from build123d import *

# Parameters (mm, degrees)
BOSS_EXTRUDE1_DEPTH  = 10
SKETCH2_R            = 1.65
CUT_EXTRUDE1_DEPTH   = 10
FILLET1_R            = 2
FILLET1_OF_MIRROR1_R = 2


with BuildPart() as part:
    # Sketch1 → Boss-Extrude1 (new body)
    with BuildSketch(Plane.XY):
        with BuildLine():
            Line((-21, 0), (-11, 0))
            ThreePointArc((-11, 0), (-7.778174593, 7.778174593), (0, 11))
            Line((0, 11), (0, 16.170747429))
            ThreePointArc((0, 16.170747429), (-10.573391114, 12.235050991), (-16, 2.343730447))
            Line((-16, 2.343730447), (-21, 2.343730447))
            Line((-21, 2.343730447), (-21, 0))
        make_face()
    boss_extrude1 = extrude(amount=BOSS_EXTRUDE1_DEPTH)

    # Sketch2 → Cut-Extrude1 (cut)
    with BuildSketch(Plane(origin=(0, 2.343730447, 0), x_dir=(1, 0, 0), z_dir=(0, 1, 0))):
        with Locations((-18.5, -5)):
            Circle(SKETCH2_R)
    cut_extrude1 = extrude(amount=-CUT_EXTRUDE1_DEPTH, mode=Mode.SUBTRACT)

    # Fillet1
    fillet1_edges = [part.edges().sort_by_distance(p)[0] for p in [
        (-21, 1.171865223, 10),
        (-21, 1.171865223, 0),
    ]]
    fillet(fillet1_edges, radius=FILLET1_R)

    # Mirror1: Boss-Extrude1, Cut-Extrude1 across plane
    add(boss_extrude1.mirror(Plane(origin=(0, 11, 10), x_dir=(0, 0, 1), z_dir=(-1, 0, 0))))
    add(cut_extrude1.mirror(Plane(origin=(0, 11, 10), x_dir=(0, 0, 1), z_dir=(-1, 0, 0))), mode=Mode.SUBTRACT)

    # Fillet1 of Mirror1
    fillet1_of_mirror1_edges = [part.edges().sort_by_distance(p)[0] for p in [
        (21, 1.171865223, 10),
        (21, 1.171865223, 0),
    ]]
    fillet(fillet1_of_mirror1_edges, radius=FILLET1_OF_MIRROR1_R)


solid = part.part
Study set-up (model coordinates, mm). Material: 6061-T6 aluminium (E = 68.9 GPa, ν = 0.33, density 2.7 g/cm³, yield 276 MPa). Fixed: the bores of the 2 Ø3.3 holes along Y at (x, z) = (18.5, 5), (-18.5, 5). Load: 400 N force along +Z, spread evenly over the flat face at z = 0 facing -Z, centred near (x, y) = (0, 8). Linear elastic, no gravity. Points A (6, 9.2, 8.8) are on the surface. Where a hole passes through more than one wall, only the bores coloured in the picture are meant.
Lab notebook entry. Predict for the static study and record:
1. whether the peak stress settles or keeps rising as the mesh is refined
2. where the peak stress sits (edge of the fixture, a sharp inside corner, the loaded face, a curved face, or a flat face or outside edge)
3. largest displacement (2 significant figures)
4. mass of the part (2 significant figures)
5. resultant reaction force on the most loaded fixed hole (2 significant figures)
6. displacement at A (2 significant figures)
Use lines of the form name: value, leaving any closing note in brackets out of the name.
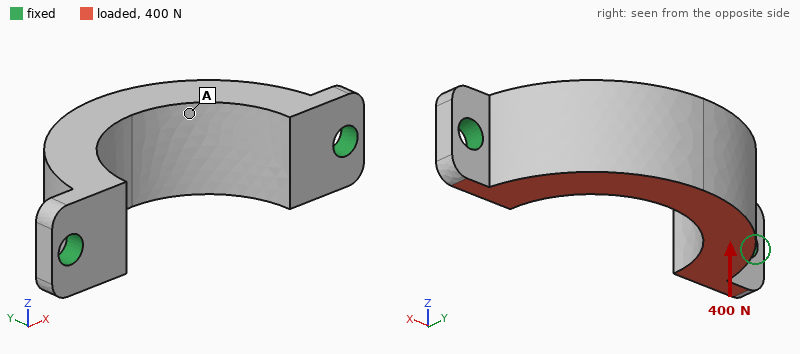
whether the peak stress settles or keeps rising as the mesh is refined: keeps rising
where the peak stress sits: edge of the fixture
largest displacement: 52 µm
mass of the part: 6.4 g
resultant reaction force on the most loaded fixed hole: 200 N
displacement at A: 30 µm
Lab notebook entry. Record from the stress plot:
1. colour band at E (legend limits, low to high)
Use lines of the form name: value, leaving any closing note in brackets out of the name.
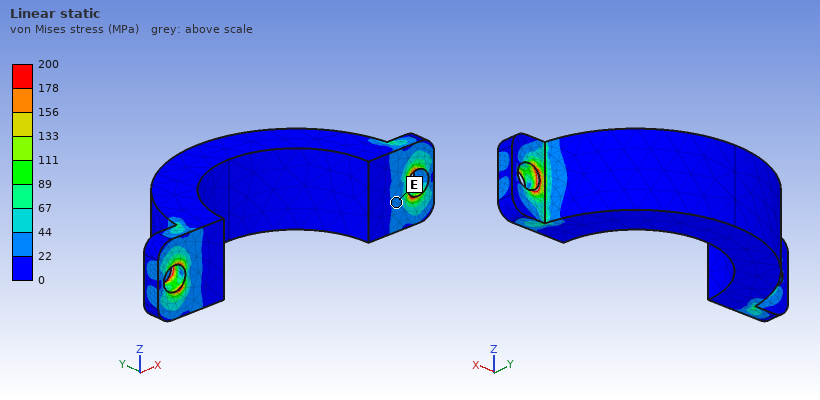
colour band at E: 22 to 44 MPa
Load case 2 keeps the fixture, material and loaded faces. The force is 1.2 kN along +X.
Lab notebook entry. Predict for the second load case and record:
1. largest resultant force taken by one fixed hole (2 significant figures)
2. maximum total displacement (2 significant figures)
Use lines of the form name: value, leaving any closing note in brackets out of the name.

largest resultant force taken by one fixed hole: 660 N
maximum total displacement: 23 µm
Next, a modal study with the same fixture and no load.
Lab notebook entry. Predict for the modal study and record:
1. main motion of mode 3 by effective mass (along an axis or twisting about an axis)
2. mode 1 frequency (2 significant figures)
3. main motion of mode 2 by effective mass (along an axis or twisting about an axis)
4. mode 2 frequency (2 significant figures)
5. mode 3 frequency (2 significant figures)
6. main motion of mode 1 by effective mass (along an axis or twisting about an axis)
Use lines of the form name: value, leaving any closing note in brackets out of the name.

main motion of mode 3 by effective mass: twisting about Y
mode 1 frequency: 6700 Hz
main motion of mode 2 by effective mass: along X
mode 2 frequency: 19 kHz
mode 3 frequency: 25 kHz
main motion of mode 1 by effective mass: along Z
